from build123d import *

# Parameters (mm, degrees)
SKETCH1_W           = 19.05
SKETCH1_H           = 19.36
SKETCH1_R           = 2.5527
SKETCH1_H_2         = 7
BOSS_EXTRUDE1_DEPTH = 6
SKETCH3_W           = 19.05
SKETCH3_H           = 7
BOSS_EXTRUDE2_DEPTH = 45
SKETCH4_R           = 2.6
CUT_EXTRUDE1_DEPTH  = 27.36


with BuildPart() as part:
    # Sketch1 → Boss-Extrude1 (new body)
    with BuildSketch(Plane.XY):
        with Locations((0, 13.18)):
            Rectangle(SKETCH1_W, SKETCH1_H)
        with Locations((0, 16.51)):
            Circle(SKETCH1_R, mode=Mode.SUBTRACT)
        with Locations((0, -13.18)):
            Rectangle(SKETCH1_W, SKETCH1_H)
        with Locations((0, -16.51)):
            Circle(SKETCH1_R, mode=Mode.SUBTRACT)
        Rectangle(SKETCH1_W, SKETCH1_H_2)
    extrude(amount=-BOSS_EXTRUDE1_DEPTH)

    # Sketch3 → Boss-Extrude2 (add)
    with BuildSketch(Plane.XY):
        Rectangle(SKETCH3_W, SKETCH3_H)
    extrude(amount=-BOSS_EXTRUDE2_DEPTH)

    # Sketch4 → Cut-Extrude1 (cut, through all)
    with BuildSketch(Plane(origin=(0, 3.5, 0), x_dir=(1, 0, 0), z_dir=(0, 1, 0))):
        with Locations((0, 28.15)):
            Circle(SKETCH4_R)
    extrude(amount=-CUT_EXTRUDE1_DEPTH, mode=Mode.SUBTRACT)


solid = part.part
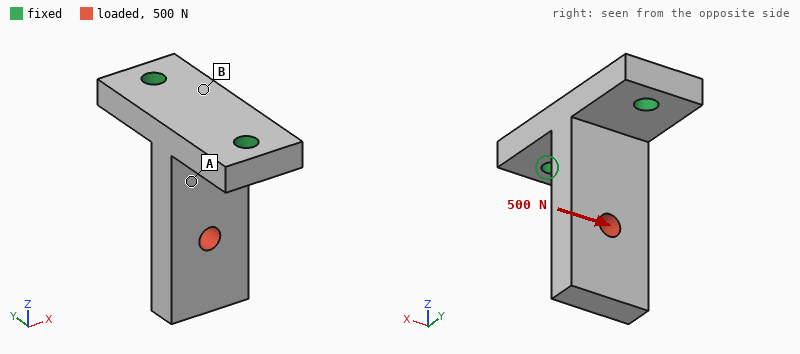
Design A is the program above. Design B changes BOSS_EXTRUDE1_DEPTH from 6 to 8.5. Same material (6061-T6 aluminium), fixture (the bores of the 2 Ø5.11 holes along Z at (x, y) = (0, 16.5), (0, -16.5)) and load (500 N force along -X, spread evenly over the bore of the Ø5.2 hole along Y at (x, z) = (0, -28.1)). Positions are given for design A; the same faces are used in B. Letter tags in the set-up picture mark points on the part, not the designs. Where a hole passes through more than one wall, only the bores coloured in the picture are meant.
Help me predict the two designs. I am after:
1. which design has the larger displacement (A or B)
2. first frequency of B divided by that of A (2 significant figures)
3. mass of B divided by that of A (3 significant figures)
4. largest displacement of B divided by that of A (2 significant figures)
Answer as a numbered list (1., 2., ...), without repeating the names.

1. A
2. 1.2
3. 1.17
4. 0.49
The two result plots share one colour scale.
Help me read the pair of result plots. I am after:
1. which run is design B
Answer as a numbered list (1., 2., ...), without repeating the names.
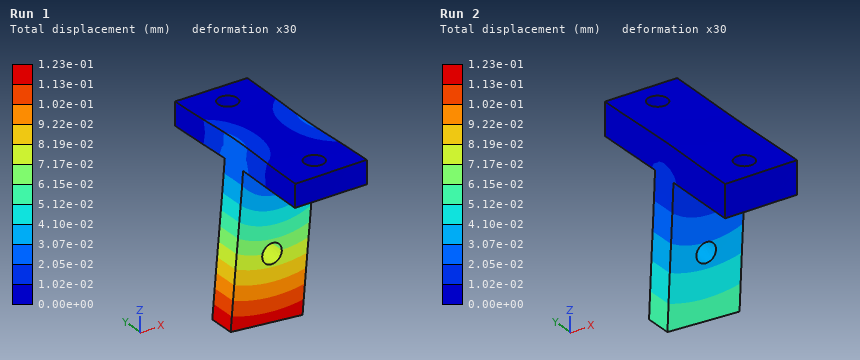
1. Run 2
